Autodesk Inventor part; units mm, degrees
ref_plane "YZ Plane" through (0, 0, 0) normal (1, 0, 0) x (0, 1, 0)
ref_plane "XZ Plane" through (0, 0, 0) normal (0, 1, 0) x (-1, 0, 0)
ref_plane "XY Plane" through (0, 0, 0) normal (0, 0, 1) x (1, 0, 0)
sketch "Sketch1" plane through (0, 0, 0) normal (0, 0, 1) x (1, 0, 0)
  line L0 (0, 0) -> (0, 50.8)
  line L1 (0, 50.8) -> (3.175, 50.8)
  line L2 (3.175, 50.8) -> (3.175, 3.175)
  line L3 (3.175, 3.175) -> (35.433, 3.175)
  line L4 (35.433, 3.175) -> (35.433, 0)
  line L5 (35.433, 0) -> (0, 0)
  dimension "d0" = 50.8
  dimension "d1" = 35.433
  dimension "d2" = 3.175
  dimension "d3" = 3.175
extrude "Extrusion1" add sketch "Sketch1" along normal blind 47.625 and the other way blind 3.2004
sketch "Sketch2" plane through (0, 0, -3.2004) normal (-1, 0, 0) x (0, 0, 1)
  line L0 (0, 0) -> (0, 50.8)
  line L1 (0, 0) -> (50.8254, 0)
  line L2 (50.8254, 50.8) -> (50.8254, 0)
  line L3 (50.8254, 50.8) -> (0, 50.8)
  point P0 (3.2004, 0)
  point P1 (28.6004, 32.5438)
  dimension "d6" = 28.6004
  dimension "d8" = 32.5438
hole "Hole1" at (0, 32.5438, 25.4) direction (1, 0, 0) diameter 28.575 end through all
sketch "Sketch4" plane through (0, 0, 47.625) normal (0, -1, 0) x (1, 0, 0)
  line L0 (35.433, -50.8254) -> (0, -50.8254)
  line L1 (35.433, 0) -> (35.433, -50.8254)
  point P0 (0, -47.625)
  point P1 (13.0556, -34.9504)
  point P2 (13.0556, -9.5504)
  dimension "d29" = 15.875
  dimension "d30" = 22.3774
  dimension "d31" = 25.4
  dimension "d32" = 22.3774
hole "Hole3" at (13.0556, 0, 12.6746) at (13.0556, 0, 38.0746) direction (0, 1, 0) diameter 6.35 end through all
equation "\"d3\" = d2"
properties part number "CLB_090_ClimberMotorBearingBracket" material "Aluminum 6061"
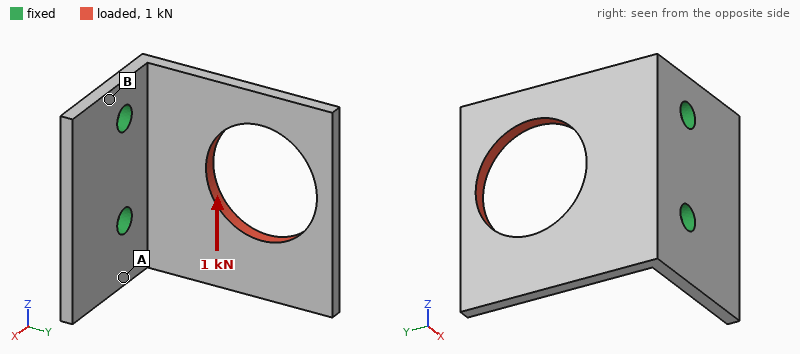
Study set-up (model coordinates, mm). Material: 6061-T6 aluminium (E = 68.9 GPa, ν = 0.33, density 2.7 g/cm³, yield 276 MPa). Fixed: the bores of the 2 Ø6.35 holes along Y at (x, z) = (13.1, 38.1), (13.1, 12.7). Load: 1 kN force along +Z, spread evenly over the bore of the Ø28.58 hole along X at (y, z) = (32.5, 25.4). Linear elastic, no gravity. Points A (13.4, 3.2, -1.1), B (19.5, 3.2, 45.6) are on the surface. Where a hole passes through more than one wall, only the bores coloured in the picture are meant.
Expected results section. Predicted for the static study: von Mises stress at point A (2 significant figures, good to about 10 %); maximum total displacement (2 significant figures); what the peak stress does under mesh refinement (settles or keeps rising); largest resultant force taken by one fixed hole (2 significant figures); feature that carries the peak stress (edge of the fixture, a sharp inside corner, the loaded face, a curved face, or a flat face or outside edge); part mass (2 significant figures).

62 MPa
0.35 mm
keeps rising
1.2 kN
edge of the fixture
30 g
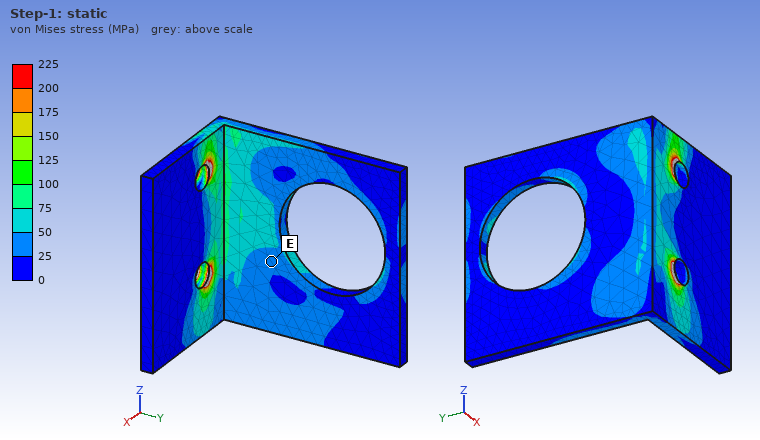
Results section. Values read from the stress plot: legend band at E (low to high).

25 to 50 MPa
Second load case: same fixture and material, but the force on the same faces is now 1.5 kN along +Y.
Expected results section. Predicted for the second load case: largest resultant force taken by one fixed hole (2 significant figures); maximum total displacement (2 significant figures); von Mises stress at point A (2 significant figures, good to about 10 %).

760 N
0.42 mm
40 MPa
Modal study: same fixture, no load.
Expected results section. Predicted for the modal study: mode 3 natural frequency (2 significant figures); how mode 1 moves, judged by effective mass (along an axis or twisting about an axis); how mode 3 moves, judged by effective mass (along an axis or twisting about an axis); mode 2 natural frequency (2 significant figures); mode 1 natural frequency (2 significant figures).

3300 Hz
along X
along Z
1900 Hz
930 Hz
